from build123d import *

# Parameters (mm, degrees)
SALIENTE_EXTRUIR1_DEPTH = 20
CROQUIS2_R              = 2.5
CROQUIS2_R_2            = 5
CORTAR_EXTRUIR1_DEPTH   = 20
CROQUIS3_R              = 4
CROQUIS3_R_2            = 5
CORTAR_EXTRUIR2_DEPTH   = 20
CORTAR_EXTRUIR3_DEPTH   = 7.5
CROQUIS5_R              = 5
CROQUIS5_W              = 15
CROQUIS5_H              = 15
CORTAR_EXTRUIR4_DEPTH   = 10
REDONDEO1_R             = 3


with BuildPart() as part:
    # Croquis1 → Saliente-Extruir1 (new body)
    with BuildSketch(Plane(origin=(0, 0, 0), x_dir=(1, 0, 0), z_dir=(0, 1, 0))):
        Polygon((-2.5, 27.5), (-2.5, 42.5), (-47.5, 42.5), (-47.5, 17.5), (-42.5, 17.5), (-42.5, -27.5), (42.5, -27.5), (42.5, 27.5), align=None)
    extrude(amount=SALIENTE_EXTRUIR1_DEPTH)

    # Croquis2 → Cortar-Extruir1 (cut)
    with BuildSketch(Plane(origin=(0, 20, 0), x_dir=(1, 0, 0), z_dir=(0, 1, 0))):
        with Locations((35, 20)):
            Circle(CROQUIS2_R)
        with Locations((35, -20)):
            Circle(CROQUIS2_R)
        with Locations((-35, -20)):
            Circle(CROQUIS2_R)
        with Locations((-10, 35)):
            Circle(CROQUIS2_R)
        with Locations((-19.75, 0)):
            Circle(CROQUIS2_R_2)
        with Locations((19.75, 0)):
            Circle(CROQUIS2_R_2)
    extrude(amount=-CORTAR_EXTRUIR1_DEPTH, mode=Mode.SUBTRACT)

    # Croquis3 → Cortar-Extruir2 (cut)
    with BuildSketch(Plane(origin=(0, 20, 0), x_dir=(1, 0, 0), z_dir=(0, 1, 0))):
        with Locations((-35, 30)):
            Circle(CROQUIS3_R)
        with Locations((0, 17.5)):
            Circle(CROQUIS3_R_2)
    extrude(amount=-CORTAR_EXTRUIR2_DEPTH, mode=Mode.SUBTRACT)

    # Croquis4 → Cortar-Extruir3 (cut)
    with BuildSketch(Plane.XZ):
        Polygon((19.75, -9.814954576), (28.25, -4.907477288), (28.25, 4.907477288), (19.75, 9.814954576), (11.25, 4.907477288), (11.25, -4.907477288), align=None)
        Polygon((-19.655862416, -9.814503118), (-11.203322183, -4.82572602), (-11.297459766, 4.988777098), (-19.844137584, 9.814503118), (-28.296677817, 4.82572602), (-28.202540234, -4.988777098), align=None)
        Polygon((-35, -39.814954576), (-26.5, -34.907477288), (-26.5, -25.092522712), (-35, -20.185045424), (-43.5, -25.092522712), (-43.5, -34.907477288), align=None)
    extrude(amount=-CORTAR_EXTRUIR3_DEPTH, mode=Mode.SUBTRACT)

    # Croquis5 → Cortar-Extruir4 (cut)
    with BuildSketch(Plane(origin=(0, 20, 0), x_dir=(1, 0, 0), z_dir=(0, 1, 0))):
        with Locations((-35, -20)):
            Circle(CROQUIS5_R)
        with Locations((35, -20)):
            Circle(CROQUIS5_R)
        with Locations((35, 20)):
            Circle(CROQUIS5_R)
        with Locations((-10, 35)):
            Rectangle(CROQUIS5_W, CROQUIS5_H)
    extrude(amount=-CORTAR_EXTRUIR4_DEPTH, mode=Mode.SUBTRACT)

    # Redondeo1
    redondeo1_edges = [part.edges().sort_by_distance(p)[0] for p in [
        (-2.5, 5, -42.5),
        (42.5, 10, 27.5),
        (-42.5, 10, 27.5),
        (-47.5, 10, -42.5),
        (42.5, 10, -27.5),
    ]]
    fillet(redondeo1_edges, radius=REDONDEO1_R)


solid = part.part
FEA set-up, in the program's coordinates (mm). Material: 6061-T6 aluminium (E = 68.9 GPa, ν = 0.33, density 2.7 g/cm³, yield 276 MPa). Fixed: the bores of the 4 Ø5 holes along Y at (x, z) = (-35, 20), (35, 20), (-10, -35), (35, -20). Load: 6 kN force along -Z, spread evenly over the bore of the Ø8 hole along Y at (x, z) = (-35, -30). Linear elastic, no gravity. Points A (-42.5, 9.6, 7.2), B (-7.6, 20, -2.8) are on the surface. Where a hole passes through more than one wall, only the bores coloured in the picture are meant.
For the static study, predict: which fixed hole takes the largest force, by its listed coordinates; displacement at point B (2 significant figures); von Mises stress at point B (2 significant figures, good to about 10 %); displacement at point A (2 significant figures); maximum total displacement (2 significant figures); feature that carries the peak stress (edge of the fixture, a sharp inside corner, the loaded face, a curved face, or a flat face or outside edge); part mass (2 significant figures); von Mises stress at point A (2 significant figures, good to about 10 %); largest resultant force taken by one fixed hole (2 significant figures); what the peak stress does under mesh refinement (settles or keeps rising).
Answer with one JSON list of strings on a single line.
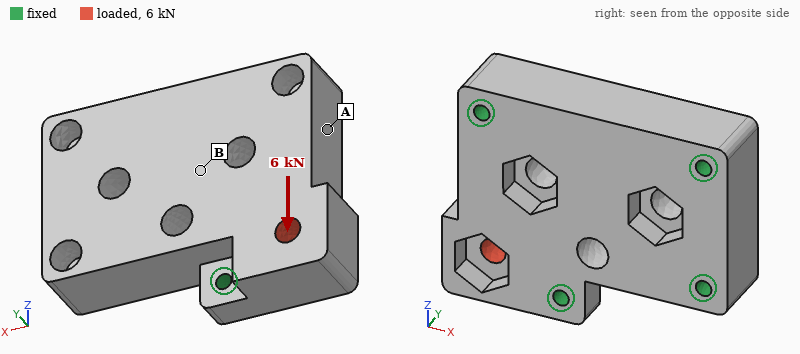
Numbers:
["(-35, 20)", "3.5 µm", "5.6 MPa", "3.5 µm", "17 µm", "edge of the fixture", "250 g", "16 MPa", "3.4 kN", "keeps rising"]
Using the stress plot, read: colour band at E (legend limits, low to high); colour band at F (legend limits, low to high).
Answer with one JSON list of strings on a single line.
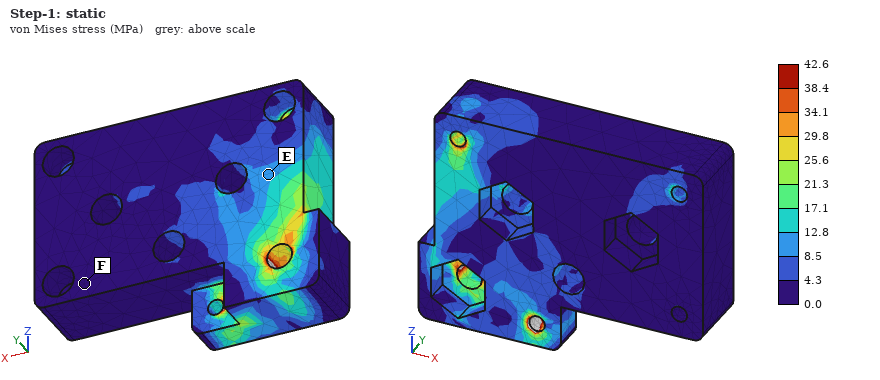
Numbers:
["8.5 to 12.8 MPa", "0.0 to 4.3 MPa"]
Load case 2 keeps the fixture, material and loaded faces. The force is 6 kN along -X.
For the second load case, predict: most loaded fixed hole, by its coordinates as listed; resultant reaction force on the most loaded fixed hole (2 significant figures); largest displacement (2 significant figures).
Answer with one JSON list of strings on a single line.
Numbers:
["(-10, -35)", "3.5 kN", "34 µm"]
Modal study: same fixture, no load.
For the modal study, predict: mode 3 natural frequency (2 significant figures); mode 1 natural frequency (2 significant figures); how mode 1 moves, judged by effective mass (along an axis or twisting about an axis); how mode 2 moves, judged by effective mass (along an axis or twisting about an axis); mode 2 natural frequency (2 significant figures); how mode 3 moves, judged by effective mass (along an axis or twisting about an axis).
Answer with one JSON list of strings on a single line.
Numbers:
["15 kHz", "7800 Hz", "along Y", "along Y", "11 kHz", "along Z"]
